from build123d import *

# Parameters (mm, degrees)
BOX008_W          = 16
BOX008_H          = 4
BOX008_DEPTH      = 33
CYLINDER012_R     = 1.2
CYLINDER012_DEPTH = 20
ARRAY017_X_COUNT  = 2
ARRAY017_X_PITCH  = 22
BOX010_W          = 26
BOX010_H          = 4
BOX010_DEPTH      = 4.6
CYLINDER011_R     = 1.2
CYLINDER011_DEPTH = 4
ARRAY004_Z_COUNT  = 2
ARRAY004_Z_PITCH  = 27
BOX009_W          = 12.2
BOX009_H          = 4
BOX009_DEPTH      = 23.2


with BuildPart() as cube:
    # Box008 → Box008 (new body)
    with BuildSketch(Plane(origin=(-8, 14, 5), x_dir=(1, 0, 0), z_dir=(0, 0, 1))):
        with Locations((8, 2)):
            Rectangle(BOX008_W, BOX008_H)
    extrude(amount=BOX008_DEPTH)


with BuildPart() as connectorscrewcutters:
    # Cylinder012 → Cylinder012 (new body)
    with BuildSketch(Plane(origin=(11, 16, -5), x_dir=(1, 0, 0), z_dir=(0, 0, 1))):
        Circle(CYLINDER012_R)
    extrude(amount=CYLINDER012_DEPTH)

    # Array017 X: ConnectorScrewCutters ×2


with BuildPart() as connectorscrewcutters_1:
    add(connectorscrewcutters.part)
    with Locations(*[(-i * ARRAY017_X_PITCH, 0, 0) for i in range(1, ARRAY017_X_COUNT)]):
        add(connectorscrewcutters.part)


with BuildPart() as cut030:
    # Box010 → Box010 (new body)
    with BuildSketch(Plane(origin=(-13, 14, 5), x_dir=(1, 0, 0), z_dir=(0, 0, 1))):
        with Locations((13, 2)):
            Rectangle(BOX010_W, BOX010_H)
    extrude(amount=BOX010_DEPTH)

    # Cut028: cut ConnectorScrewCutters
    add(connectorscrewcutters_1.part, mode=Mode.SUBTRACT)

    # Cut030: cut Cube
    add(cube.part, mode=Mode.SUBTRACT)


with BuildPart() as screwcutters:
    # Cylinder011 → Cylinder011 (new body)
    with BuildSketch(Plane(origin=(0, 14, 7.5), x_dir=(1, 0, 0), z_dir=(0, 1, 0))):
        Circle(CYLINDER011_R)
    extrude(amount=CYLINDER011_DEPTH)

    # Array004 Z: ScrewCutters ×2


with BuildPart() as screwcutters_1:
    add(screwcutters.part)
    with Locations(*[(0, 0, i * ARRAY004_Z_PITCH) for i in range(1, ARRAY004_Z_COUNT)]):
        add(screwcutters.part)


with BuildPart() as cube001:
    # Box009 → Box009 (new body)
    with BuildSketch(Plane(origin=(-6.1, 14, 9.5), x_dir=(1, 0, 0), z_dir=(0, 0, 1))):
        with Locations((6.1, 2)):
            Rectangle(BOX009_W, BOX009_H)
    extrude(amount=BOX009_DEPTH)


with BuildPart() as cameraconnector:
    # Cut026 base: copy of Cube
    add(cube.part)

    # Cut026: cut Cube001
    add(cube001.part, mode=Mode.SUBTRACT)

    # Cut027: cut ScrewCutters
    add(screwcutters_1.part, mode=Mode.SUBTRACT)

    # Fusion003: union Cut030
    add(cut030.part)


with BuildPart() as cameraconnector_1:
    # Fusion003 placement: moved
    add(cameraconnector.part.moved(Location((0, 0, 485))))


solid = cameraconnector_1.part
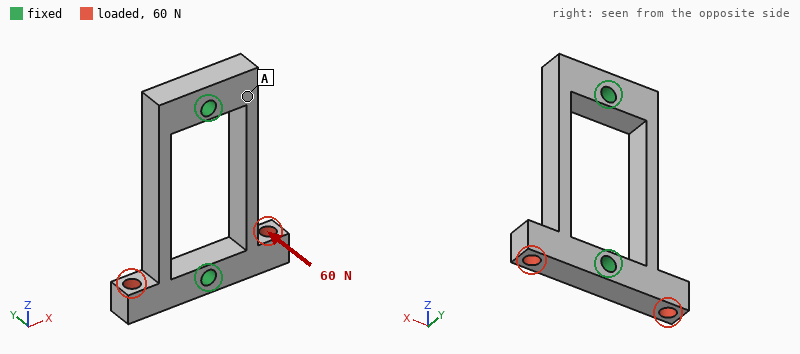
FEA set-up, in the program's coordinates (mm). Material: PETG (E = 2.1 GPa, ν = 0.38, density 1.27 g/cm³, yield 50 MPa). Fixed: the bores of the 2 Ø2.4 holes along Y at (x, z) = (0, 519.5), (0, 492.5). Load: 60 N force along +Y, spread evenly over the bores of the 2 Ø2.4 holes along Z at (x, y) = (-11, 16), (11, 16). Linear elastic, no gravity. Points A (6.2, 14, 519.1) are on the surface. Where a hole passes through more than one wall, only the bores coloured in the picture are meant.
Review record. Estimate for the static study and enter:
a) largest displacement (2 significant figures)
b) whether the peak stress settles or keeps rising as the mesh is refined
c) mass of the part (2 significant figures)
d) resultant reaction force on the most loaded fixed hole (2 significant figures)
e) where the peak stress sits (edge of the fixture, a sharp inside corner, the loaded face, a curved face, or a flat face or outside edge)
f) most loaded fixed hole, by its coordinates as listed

0.32 mm
keeps rising
1.4 g
59 N
edge of the fixture
(0, 492.5)
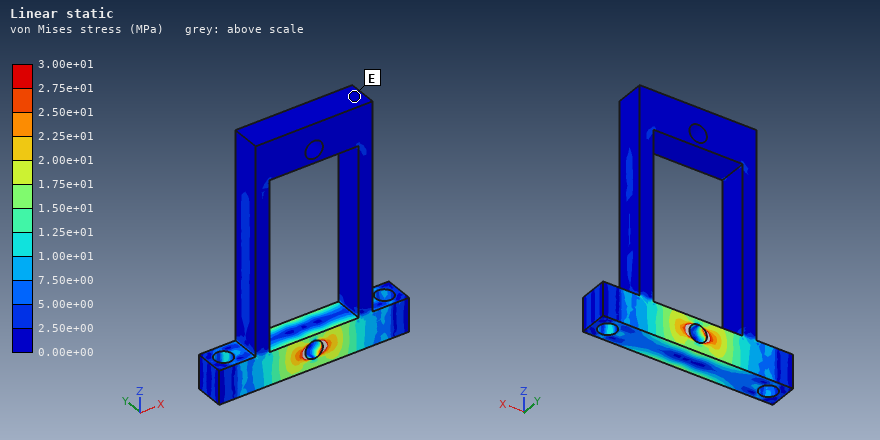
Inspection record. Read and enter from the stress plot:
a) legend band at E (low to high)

0.00e+00 to 2.50e+00 MPa
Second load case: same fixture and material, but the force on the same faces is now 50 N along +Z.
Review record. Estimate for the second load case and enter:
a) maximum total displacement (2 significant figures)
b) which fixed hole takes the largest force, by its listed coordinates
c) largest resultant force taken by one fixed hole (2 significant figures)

0.15 mm
(0, 519.5)
34 N
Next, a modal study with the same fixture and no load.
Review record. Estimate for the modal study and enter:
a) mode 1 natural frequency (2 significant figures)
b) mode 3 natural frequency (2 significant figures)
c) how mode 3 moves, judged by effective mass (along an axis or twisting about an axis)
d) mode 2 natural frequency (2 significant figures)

3800 Hz
4400 Hz
twisting about Z
3800 Hz
